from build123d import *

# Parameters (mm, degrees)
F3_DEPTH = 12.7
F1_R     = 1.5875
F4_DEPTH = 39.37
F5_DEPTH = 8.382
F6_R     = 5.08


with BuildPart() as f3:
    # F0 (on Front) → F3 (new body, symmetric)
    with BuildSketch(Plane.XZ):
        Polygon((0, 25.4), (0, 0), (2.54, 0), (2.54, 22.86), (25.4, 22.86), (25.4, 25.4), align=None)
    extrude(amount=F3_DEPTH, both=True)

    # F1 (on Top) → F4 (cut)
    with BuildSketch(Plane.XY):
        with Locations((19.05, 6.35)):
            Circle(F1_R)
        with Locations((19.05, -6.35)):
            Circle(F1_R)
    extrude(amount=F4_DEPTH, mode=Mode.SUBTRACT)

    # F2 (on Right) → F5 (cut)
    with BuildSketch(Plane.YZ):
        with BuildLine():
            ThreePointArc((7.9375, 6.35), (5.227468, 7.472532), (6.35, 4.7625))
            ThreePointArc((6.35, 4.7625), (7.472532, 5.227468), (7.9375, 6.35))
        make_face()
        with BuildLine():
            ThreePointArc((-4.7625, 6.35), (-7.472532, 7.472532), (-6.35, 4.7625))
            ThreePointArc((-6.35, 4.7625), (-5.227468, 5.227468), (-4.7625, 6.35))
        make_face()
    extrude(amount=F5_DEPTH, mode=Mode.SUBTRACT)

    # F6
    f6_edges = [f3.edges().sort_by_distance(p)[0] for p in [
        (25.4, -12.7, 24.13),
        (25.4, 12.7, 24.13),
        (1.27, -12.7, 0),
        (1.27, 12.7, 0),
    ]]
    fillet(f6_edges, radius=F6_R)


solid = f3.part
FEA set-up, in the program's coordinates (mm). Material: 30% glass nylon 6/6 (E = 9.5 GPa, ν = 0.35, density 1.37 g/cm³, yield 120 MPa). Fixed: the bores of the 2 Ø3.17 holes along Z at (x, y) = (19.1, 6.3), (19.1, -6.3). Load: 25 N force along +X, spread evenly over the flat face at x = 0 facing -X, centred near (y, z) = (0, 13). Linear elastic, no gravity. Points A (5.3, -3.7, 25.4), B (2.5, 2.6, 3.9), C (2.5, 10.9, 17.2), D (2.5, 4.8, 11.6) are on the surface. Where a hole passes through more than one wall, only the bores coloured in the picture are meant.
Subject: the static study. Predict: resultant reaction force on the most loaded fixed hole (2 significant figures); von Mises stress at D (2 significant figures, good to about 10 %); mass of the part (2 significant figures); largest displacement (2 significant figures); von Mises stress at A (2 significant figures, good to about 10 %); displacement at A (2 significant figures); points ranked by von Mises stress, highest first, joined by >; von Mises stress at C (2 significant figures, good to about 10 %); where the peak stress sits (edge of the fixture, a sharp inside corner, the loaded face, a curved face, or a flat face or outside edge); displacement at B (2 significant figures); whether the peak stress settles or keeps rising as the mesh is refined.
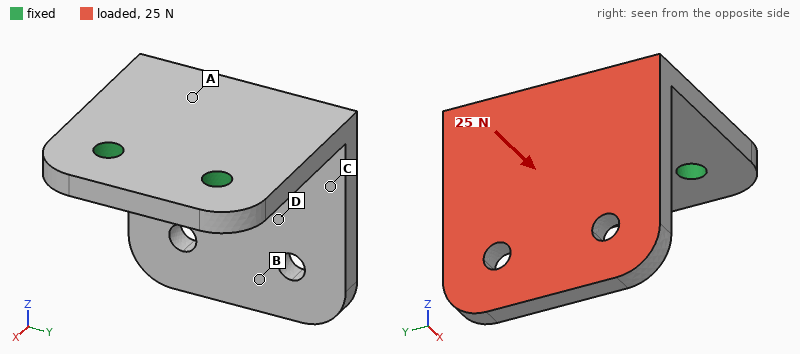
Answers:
13 N
2.1 MPa
4.1 g
0.45 mm
8.8 MPa
0.071 mm
A > C > D > B
4.6 MPa
edge of the fixture
0.36 mm
keeps rising
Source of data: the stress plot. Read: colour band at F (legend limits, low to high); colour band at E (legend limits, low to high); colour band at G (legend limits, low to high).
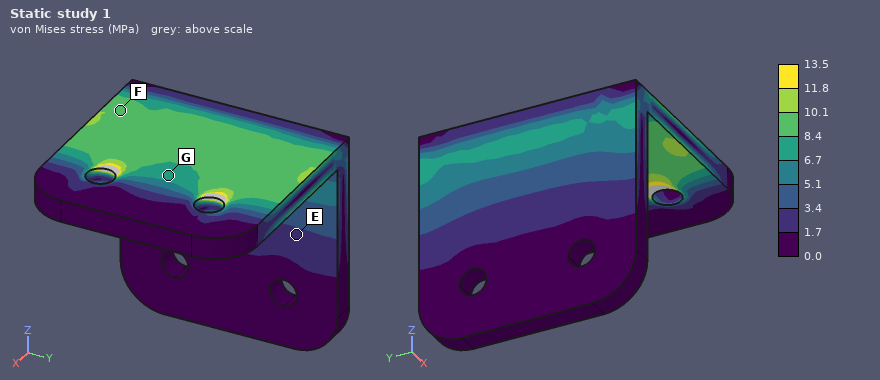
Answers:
8.4 to 10.1 MPa
1.7 to 3.4 MPa
6.7 to 8.4 MPa
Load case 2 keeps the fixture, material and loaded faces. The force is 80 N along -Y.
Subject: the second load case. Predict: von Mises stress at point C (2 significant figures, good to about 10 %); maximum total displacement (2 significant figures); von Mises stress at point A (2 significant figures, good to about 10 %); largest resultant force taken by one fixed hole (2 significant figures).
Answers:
7.9 MPa
0.46 mm
14 MPa
120 N
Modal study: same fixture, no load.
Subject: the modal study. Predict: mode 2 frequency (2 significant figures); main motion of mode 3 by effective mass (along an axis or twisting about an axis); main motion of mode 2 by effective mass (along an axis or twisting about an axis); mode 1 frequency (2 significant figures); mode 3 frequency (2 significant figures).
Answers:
1600 Hz
along Z
along Y
890 Hz
2500 Hz
